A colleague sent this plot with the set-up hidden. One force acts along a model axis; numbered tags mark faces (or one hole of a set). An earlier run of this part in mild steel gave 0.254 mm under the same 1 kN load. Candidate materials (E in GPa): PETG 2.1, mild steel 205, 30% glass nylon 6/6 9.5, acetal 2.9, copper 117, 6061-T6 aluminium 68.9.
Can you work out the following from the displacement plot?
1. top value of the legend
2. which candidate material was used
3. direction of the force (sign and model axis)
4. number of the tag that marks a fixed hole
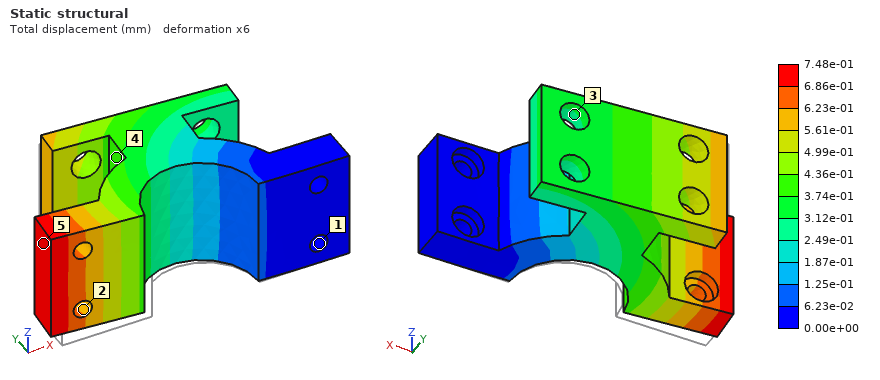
7.48e-01 mm
6061-T6 aluminium
+Y
1
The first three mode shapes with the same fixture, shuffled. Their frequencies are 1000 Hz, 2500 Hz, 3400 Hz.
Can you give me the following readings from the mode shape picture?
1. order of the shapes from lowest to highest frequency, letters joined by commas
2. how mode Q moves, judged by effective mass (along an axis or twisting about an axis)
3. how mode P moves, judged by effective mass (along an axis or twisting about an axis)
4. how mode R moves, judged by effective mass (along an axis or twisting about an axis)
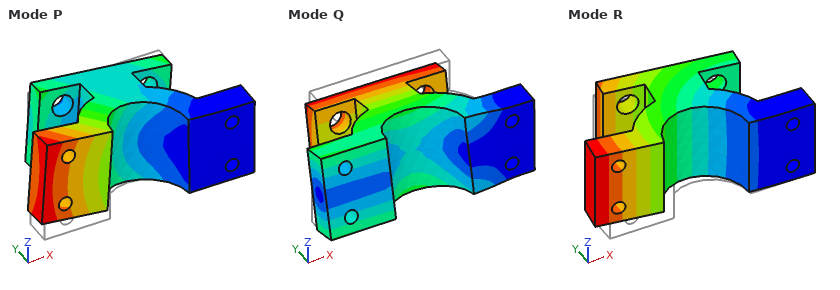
R, P, Q
along Z
along Z
along Y
